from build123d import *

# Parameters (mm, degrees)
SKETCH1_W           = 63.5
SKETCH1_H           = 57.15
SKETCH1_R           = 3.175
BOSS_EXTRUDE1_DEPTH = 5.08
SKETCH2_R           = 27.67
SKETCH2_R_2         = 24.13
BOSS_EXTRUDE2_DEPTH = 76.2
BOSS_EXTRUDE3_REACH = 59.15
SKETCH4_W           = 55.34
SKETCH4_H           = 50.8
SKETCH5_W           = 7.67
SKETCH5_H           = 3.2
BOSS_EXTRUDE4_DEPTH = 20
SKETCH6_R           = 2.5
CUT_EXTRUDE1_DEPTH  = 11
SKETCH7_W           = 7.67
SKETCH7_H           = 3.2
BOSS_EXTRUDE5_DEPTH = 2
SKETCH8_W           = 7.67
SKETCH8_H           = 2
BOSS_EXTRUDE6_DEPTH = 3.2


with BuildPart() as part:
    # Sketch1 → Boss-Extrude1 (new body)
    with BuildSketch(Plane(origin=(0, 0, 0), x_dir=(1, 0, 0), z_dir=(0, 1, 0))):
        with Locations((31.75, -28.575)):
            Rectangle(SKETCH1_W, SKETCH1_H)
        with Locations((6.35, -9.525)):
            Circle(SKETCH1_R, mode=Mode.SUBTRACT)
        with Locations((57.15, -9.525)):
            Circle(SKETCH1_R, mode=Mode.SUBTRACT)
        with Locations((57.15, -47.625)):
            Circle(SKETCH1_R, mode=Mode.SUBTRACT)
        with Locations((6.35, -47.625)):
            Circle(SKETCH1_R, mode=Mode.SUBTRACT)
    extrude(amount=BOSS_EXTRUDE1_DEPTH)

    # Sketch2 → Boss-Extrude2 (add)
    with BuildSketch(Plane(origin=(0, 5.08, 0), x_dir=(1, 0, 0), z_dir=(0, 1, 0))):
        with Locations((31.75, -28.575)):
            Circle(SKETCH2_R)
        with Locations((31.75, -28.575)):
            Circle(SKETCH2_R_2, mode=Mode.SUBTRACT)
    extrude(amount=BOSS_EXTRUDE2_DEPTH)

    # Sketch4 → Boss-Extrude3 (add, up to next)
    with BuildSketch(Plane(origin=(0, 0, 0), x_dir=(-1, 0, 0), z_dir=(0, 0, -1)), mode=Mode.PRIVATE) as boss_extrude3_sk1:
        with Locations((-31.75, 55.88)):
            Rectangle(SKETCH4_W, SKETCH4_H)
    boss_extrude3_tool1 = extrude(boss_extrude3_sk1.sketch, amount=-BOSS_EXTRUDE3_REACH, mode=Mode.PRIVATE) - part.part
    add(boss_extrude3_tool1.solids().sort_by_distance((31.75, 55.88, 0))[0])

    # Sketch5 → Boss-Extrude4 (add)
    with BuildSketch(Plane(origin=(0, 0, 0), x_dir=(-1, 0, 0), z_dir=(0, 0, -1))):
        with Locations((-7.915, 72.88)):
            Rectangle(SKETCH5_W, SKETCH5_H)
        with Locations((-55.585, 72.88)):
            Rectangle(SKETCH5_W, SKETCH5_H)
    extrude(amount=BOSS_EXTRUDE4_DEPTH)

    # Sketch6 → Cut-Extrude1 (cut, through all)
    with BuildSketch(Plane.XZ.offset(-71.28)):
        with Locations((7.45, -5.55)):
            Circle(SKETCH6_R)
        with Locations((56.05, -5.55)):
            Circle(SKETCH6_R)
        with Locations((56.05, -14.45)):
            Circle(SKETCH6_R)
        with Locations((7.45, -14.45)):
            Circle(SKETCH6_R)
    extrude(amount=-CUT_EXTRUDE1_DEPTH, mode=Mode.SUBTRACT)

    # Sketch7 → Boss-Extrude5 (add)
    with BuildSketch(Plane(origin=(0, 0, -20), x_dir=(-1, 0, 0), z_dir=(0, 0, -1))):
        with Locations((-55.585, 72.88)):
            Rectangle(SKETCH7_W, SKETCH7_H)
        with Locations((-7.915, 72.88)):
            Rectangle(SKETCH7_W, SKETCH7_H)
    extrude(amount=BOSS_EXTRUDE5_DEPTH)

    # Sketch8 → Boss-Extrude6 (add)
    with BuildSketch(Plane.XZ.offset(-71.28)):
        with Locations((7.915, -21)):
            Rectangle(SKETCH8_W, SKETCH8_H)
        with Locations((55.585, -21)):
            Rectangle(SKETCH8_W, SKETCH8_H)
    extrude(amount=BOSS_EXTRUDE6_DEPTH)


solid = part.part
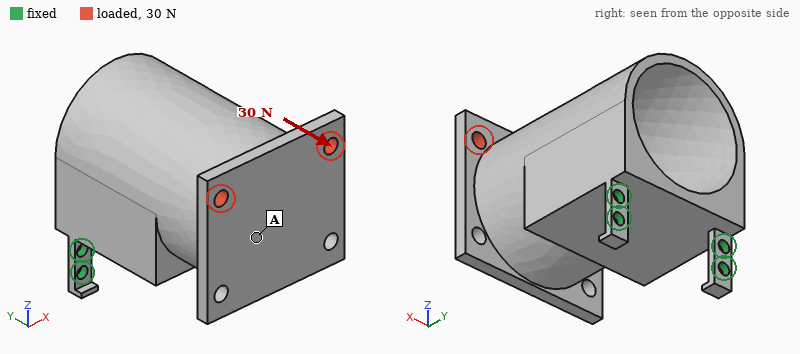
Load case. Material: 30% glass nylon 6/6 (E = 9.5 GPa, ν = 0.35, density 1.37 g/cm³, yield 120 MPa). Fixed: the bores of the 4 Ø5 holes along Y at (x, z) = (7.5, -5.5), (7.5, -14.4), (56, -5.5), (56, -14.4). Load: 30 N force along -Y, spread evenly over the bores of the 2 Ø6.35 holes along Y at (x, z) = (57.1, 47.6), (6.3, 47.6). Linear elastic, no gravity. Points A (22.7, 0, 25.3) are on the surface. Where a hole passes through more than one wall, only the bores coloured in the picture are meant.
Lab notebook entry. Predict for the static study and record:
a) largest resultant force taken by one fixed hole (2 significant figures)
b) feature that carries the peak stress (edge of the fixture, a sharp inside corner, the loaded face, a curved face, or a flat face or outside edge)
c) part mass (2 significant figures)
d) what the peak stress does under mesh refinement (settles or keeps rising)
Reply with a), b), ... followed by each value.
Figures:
a) 16 N
b) edge of the fixture
c) 110 g
d) keeps rising
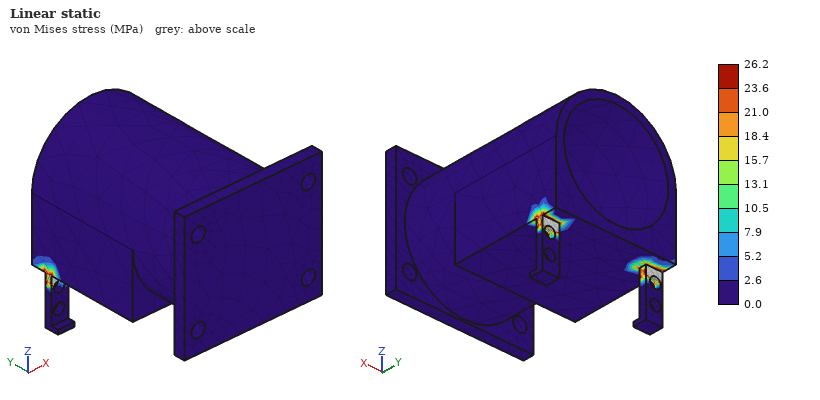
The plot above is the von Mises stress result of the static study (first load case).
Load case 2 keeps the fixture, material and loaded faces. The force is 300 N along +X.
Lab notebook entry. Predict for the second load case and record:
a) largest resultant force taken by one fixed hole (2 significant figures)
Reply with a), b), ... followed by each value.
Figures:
a) 550 N
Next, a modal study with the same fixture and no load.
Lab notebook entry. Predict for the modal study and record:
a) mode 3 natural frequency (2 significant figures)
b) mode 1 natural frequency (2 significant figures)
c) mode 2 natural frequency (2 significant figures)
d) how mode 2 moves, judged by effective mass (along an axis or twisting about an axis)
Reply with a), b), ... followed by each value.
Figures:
a) 1200 Hz
b) 85 Hz
c) 810 Hz
d) along X
